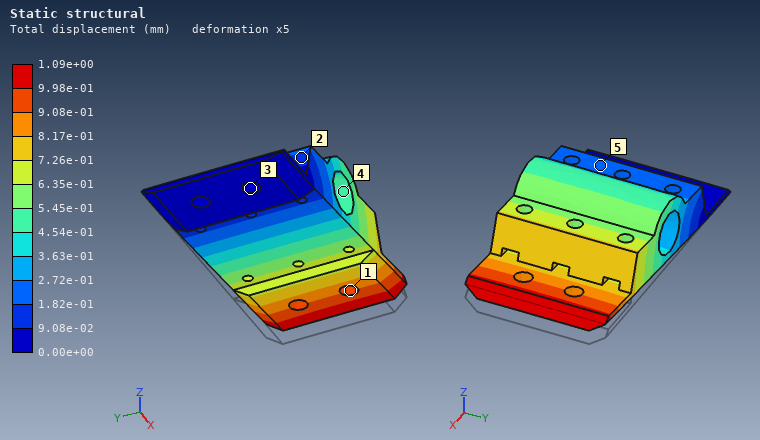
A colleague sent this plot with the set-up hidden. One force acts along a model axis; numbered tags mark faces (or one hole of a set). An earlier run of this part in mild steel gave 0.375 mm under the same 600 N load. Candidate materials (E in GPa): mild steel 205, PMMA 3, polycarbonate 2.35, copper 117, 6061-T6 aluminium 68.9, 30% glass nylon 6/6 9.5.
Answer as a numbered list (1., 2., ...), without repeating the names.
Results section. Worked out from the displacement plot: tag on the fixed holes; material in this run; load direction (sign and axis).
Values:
1. 3
2. 6061-T6 aluminium
3. +Z
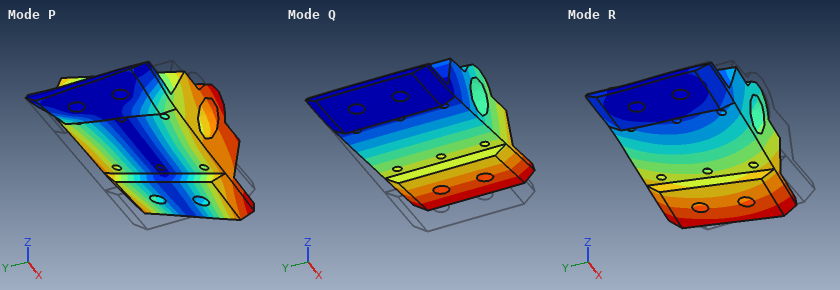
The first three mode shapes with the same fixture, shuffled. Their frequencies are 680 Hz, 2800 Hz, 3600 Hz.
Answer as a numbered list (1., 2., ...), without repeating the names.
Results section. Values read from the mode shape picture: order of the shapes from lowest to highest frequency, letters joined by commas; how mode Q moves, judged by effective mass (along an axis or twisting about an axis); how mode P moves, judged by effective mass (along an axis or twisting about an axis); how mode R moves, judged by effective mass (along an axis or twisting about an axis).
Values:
1. Q, R, P
2. along Z
3. along Y
4. along Y
